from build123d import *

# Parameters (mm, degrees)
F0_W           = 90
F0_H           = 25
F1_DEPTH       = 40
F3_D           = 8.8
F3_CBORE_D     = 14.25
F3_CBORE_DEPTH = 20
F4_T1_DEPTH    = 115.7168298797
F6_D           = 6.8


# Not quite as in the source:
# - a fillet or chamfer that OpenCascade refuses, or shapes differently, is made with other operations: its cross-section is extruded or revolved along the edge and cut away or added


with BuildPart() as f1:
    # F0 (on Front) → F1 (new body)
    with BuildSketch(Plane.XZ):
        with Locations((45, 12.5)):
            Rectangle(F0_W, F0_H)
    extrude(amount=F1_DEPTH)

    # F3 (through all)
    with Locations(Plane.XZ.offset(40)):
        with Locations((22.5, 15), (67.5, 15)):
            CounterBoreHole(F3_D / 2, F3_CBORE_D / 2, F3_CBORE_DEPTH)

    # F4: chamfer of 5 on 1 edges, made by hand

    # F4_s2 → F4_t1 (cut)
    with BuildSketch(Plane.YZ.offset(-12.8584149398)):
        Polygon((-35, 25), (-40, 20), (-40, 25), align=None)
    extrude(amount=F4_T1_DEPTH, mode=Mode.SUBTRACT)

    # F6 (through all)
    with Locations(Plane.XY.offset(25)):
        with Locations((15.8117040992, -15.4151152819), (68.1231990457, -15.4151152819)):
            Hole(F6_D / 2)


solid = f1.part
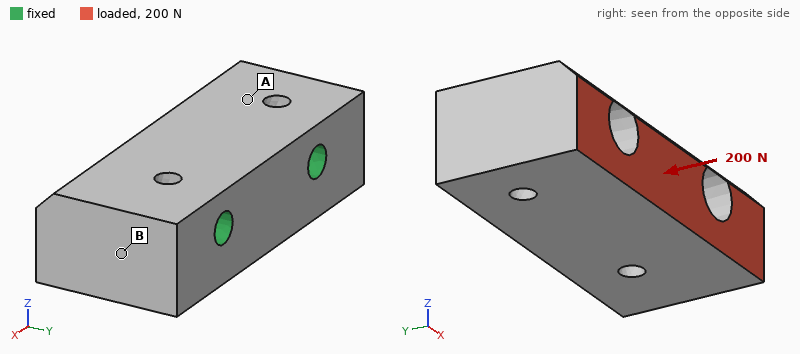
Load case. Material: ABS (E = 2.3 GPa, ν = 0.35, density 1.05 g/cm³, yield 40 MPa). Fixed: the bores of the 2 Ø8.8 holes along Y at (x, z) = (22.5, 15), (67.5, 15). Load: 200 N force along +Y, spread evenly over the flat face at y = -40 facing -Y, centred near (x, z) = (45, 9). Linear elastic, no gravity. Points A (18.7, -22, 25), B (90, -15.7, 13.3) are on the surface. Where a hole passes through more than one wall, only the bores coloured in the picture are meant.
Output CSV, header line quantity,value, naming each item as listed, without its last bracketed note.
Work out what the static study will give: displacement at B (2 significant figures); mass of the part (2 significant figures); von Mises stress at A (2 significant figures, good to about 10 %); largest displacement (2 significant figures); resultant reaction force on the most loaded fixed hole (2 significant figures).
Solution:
quantity,value
displacement at B,2.6 µm
mass of the part,83 g
von Mises stress at A,0.18 MPa
largest displacement,7.4 µm
resultant reaction force on the most loaded fixed hole,100 N
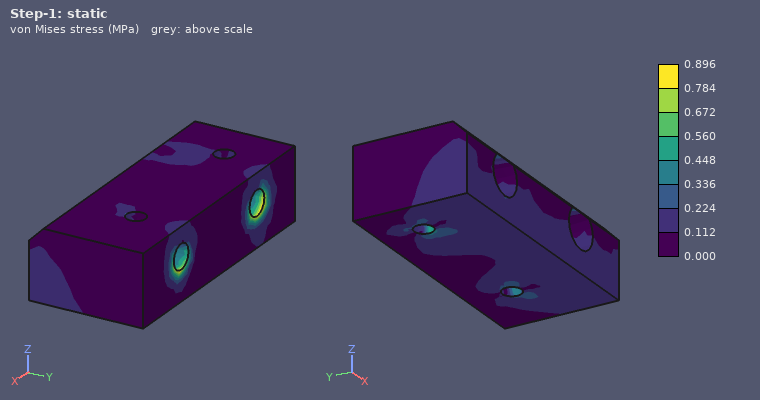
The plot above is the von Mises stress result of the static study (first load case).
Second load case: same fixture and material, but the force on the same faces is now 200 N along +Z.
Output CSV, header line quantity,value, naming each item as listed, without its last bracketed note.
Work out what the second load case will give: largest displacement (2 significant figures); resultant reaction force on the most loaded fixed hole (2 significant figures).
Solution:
quantity,value
largest displacement,30 µm
resultant reaction force on the most loaded fixed hole,100 N
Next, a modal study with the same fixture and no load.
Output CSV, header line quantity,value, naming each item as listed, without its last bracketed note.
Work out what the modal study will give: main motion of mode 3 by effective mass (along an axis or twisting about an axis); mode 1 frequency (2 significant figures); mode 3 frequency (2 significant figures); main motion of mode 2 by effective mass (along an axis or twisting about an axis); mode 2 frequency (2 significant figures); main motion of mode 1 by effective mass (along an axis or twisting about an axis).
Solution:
quantity,value
main motion of mode 3 by effective mass,along X
mode 1 frequency,3000 Hz
mode 3 frequency,4200 Hz
main motion of mode 2 by effective mass,twisting about Y
mode 2 frequency,3500 Hz
main motion of mode 1 by effective mass,along Z
